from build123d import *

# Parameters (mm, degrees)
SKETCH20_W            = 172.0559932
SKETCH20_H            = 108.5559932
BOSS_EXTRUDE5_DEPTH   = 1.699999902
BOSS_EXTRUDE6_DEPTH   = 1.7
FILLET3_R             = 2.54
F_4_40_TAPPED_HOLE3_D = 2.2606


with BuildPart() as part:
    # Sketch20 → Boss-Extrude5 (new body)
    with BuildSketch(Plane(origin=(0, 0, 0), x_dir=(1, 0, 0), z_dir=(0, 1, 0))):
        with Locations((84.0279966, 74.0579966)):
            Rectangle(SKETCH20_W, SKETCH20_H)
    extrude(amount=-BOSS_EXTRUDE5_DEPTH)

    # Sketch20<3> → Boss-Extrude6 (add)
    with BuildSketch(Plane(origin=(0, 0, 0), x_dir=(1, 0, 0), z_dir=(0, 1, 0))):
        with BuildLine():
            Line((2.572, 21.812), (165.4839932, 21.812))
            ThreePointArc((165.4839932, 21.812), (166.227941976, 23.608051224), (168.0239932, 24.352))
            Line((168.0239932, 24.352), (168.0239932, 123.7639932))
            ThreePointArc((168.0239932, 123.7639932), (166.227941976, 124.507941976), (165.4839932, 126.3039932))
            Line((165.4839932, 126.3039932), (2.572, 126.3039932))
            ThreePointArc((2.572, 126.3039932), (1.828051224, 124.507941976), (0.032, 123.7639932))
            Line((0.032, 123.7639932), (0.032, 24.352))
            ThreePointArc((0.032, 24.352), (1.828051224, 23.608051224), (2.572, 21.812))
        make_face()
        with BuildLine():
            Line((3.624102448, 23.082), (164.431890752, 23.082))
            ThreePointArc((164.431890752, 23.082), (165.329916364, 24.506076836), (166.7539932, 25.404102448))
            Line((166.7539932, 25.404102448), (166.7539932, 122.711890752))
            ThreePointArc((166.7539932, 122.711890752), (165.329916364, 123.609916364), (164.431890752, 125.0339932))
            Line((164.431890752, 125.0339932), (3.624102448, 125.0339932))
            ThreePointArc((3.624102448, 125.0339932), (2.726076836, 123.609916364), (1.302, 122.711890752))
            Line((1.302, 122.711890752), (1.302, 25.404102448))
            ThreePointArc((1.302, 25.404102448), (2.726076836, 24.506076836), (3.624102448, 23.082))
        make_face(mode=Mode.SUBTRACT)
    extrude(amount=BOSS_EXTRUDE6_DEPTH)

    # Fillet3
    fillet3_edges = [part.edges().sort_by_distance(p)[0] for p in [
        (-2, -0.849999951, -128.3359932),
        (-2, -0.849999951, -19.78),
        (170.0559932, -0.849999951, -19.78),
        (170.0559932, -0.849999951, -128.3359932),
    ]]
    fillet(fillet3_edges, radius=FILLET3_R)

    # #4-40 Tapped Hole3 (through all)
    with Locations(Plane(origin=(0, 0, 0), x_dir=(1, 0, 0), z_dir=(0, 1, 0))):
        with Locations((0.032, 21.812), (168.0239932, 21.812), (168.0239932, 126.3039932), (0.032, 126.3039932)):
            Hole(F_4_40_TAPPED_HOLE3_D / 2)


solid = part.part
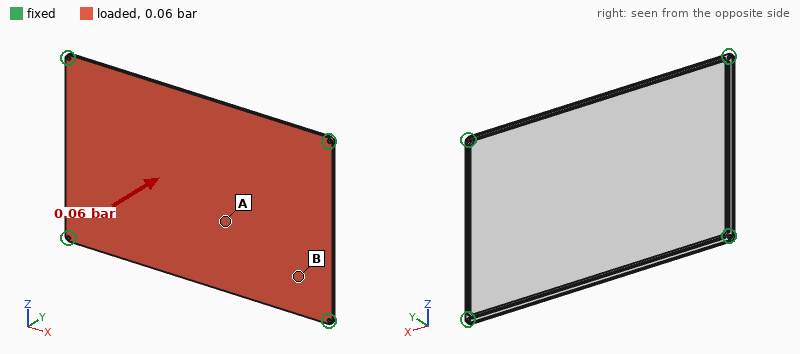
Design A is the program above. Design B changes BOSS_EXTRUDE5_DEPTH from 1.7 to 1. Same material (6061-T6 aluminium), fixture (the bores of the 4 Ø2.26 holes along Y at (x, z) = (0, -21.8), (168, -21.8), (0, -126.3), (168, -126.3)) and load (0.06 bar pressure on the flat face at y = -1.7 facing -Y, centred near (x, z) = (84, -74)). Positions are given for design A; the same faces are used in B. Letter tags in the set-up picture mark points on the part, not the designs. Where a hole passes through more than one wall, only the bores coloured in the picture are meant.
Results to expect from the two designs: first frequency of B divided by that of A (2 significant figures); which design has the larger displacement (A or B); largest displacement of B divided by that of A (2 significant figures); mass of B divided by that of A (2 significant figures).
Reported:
0.70
B
3.6
0.60
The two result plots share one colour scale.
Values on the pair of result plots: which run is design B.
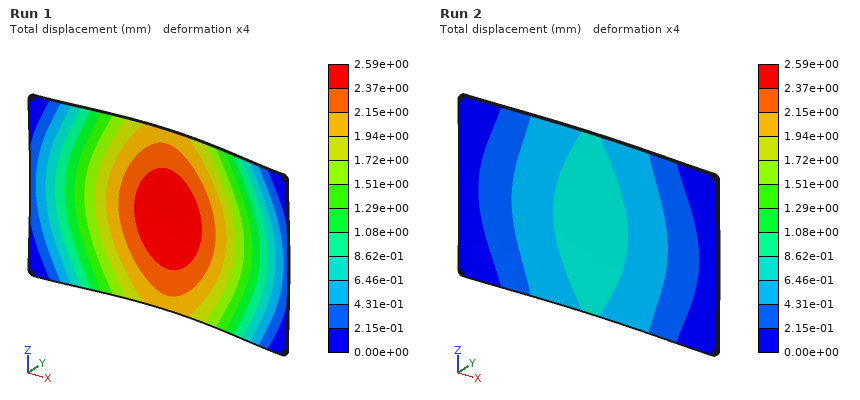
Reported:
Run 1
